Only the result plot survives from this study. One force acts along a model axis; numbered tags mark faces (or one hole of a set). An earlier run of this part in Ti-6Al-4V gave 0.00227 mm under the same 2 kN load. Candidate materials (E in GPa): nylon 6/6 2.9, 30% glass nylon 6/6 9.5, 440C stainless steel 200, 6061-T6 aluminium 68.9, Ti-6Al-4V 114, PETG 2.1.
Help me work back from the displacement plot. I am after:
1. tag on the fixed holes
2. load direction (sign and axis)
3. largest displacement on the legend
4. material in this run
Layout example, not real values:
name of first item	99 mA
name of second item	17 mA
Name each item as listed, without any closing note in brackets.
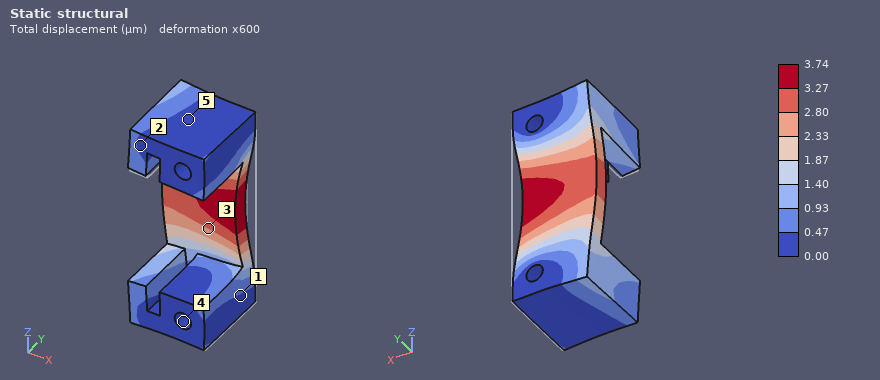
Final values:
tag on the fixed holes	4
load direction	-X
largest displacement on the legend	3.74 µm
material in this run	6061-T6 aluminium
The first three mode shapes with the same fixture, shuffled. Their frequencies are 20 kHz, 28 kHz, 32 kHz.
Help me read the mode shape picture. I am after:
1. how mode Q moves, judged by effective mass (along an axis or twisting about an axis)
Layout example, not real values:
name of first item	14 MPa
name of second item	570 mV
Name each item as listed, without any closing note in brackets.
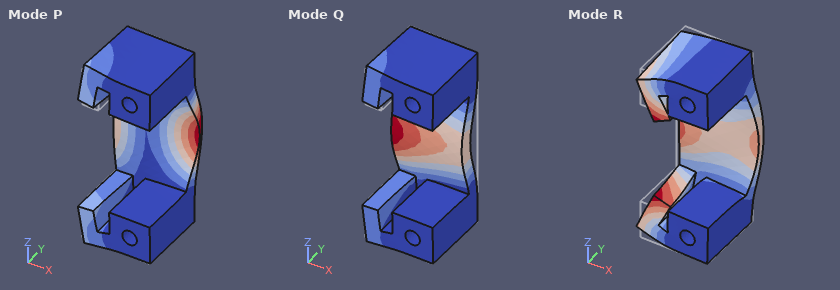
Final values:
how mode Q moves, judged by effective mass	along Y
